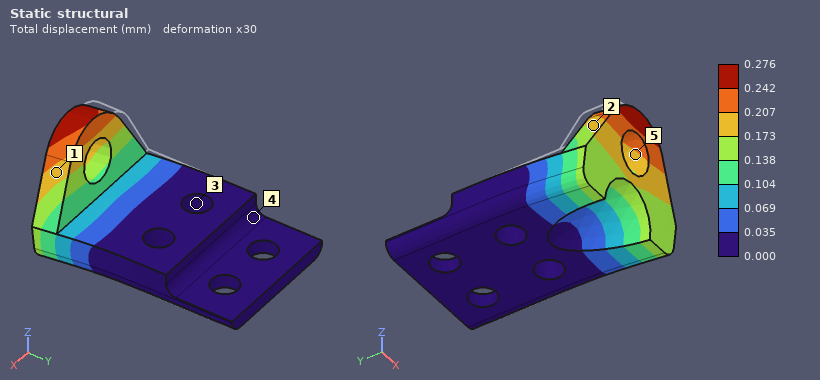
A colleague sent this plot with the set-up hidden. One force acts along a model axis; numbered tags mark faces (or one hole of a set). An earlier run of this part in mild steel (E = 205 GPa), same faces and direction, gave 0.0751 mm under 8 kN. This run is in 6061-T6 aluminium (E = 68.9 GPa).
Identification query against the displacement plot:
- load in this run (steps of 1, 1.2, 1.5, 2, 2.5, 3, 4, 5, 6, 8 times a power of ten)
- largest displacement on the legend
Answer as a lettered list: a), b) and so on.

a) 10 kN
b) 0.276 mm
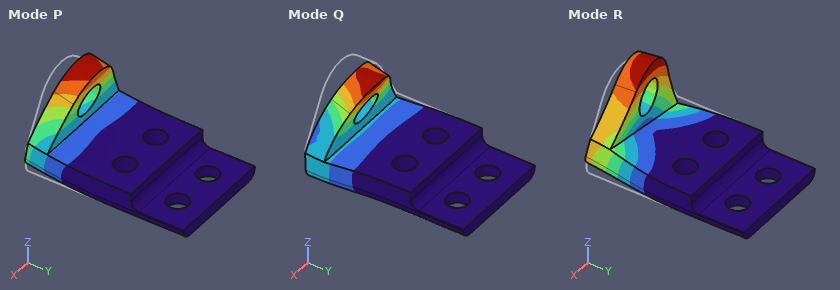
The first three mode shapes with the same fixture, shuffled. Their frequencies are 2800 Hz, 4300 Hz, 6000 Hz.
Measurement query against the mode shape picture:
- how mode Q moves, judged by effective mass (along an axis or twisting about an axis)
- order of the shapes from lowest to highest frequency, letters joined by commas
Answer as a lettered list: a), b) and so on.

a) along Z
b) P, R, Q
